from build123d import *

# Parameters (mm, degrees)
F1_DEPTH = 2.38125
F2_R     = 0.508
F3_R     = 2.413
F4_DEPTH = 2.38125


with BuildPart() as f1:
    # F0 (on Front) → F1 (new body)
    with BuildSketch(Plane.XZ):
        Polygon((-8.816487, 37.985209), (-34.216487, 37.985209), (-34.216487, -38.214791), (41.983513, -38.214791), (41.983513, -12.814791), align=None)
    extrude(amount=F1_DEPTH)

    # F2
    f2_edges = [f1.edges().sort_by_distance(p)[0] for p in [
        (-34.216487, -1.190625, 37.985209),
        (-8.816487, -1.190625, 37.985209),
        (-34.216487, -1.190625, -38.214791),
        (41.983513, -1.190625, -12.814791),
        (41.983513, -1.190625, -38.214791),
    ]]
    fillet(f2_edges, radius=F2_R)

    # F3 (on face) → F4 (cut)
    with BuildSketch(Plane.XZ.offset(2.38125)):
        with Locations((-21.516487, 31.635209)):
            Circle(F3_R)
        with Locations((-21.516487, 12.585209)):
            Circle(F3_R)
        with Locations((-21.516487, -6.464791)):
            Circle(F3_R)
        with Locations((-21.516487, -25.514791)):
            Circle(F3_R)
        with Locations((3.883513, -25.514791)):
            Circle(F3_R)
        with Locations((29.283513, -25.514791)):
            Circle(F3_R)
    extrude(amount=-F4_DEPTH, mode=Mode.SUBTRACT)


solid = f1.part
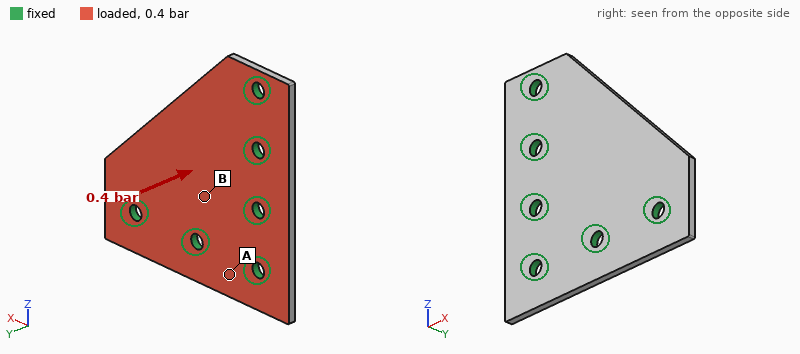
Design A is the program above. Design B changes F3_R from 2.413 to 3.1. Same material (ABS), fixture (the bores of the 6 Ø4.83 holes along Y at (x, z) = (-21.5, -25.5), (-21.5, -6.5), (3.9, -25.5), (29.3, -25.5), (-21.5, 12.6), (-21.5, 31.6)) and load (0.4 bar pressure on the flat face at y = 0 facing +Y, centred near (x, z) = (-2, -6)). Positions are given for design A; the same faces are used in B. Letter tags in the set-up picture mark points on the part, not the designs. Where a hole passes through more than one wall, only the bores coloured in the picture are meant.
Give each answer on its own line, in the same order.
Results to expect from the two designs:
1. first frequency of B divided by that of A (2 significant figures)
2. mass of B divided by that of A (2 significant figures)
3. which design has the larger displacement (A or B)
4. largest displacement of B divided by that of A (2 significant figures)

1.1
0.98
A
0.91
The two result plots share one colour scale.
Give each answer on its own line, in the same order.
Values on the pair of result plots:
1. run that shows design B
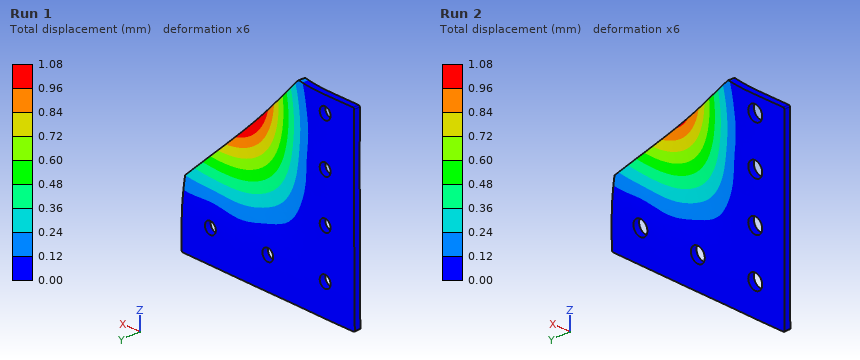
Run 2
